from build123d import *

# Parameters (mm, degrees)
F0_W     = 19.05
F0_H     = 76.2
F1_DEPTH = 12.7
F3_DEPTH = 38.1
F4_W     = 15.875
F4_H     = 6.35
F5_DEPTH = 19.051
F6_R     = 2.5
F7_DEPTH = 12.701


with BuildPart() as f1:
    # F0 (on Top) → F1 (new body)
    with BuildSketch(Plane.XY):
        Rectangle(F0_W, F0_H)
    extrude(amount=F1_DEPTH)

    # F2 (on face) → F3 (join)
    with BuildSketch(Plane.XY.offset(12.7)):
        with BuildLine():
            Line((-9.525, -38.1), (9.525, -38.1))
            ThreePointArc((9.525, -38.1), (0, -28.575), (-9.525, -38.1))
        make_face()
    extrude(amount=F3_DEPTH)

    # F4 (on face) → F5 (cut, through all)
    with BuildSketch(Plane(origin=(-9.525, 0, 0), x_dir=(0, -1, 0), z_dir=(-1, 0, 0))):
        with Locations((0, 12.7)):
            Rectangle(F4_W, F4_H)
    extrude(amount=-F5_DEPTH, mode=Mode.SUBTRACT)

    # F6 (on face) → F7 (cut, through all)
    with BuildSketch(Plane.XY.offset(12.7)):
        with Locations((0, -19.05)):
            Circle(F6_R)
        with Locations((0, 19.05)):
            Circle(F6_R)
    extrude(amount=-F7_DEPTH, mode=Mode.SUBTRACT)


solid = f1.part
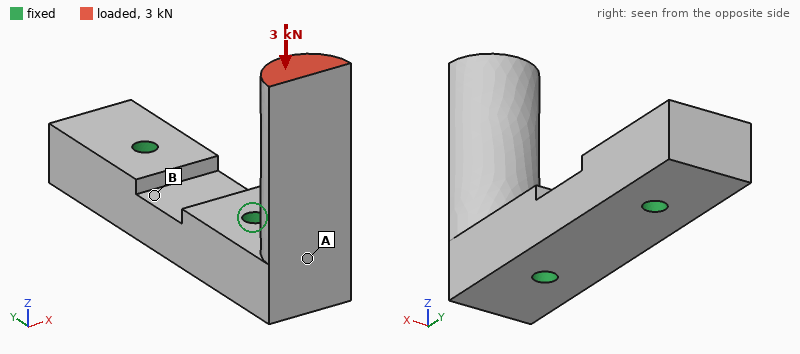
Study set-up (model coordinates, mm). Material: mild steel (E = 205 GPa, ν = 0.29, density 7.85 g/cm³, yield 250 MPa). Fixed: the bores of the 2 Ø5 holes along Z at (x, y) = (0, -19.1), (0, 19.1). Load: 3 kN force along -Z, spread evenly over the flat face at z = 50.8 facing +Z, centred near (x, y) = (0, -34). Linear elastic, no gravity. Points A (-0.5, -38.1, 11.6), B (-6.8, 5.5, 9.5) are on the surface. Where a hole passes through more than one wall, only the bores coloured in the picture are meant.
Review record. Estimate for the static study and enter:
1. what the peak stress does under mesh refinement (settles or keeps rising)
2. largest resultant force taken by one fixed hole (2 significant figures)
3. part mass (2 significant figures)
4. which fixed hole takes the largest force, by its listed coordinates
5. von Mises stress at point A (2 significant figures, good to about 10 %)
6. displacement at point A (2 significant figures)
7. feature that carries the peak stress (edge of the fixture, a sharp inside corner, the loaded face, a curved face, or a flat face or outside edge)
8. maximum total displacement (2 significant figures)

keeps rising
3.2 kN
180 g
(0, -19.1)
23 MPa
11 µm
edge of the fixture
32 µm
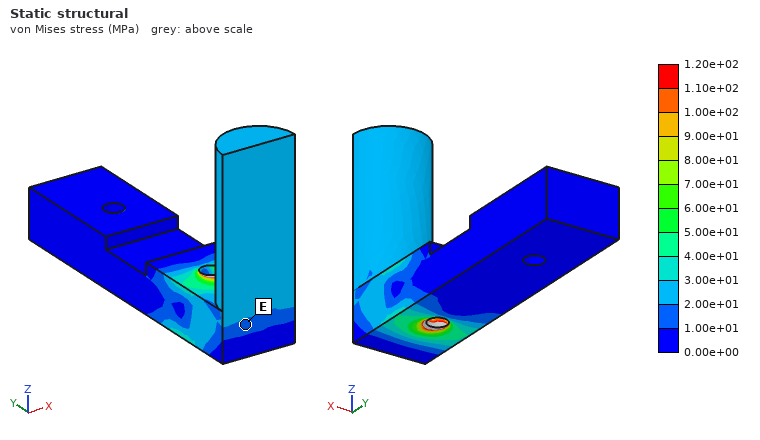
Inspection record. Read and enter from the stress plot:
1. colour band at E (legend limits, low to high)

1.00e+01 to 2.00e+01 MPa
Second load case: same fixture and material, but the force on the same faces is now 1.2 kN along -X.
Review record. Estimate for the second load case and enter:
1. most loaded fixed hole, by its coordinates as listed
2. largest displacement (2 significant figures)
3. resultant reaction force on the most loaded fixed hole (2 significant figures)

(0, -19.1)
0.11 mm
1.5 kN
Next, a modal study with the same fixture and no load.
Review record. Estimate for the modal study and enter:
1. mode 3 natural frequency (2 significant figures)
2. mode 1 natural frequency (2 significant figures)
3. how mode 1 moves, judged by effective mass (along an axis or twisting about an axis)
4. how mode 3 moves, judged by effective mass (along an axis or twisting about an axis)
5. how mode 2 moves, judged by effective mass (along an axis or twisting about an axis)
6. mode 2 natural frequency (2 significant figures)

13 kHz
3400 Hz
along Y
along Z
along X
4400 Hz
